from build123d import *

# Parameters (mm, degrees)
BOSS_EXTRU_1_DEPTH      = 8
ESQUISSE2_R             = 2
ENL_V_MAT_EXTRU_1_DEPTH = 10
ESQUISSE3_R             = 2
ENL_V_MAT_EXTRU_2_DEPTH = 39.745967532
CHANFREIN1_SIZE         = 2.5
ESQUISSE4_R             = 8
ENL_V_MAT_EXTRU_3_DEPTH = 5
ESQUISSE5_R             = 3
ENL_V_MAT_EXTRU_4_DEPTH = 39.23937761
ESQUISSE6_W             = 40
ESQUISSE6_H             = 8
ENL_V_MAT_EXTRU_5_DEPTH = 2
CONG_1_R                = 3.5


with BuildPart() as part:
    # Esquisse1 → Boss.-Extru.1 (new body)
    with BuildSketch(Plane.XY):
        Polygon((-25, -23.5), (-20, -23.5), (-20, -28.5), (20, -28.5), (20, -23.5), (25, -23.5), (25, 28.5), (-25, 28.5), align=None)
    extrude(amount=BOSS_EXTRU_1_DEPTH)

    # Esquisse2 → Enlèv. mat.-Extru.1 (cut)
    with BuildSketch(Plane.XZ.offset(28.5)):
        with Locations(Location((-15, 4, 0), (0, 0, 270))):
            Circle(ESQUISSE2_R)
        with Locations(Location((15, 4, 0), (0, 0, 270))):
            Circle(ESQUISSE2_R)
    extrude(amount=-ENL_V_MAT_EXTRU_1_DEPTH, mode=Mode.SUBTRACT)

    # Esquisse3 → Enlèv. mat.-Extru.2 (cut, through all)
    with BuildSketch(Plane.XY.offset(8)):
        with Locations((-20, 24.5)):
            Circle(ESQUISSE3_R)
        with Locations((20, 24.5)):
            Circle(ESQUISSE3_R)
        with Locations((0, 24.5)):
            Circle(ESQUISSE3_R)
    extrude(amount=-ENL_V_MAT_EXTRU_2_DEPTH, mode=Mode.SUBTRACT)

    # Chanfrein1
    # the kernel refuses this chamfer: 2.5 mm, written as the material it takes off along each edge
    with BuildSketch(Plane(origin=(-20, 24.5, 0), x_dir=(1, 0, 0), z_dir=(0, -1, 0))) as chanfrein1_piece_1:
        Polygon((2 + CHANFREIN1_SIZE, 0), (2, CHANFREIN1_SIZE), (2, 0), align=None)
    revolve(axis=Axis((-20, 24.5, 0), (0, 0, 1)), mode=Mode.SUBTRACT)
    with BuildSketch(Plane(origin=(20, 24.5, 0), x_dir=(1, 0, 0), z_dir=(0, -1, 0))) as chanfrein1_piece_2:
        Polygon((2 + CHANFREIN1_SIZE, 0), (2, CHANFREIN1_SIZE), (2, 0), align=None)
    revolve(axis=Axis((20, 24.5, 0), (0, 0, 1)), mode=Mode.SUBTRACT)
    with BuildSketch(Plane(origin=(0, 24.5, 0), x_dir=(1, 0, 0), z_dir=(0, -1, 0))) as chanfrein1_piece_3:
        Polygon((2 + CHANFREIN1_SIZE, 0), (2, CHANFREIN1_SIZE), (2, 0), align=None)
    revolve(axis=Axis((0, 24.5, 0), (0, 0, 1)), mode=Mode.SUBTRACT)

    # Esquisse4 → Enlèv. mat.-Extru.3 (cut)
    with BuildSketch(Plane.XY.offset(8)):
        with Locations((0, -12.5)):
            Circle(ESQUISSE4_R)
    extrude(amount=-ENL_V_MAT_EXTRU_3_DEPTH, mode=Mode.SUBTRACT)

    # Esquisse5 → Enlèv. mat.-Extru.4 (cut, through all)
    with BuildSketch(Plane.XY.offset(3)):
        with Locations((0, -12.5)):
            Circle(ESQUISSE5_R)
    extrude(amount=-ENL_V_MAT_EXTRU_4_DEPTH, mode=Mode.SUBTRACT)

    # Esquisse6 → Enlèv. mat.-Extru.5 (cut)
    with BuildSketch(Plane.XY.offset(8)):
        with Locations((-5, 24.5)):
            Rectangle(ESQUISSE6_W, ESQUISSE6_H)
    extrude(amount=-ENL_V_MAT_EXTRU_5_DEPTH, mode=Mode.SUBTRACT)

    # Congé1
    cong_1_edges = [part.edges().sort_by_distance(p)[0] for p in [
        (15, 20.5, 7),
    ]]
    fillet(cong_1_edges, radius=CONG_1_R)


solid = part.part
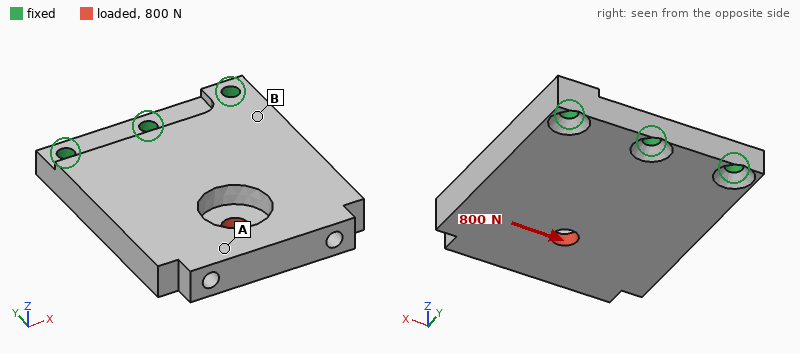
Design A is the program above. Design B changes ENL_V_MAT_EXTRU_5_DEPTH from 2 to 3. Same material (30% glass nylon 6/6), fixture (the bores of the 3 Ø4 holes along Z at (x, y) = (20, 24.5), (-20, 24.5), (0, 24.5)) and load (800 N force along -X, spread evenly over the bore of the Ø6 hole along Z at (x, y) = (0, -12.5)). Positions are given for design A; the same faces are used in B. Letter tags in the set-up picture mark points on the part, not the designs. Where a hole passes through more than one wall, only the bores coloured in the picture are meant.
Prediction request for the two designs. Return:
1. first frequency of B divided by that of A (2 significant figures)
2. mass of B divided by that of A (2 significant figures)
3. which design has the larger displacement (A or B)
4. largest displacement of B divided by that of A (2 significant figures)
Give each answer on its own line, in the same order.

0.89
0.99
B
1.5
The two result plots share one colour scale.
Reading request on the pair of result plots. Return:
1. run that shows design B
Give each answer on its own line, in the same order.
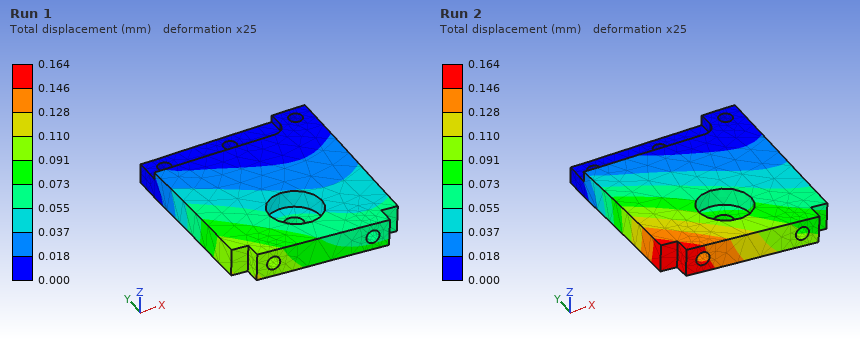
Run 2
